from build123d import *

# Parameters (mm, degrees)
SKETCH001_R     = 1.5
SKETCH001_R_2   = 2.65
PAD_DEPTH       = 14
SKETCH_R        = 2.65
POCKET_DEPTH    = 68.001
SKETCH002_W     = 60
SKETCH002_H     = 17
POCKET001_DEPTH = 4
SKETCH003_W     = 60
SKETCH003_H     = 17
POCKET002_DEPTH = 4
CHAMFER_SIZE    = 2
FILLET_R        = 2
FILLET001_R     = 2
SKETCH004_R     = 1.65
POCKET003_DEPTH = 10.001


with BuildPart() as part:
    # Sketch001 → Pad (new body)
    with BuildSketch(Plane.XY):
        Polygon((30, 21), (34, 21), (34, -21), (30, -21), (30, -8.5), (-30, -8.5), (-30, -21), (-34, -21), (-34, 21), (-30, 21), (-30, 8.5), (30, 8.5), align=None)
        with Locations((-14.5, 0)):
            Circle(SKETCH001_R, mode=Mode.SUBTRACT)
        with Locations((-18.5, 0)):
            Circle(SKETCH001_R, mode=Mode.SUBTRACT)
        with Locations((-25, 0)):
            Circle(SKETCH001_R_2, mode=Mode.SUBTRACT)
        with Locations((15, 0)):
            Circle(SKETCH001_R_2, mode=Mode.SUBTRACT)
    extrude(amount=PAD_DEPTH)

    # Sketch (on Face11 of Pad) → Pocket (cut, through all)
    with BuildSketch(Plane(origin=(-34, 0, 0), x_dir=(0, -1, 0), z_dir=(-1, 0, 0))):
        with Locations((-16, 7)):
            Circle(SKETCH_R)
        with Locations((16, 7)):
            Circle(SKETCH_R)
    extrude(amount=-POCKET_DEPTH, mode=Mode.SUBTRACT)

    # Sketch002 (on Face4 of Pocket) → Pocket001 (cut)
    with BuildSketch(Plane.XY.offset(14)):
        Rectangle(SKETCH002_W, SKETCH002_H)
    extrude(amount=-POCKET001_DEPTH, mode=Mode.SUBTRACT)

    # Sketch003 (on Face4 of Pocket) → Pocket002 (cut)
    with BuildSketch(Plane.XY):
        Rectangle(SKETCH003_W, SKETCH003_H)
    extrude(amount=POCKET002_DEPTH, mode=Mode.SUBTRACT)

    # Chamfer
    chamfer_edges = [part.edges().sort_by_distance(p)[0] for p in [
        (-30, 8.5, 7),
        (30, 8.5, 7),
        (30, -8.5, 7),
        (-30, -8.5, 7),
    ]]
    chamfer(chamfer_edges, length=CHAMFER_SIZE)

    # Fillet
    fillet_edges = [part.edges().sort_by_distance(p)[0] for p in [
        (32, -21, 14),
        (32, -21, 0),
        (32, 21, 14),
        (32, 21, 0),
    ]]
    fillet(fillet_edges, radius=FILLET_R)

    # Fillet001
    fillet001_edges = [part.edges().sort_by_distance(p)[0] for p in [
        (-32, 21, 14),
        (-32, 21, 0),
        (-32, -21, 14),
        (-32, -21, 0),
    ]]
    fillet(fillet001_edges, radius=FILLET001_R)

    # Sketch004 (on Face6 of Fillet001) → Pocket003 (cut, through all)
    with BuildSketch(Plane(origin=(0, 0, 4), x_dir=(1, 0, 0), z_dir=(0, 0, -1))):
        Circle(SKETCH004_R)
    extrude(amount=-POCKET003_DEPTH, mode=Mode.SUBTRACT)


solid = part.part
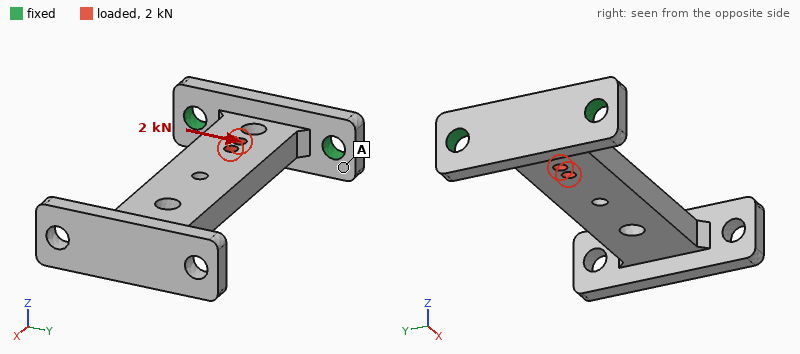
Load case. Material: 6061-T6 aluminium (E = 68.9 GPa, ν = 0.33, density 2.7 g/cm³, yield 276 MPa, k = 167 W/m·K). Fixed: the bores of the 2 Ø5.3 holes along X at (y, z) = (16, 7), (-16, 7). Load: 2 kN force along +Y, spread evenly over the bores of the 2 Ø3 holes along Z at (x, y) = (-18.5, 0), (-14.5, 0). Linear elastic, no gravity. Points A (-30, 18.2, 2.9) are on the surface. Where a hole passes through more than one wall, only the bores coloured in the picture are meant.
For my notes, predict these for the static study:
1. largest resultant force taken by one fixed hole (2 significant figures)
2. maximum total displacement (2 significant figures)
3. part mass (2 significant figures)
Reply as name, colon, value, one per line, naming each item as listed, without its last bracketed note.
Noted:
largest resultant force taken by one fixed hole: 1.6 kN
maximum total displacement: 0.17 mm
part mass: 27 g
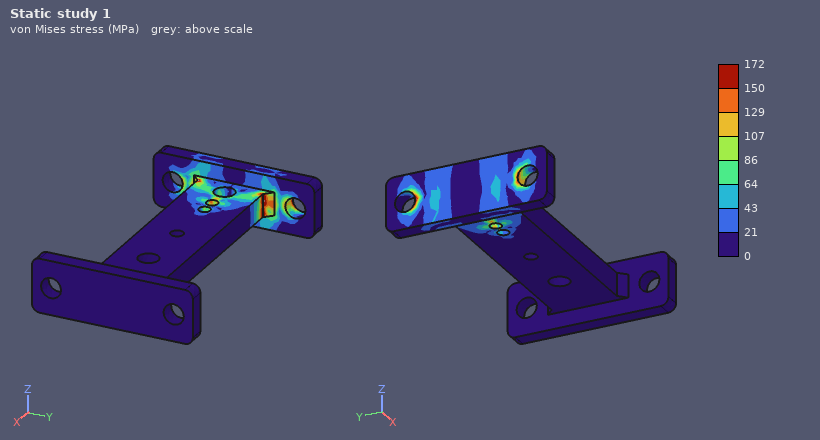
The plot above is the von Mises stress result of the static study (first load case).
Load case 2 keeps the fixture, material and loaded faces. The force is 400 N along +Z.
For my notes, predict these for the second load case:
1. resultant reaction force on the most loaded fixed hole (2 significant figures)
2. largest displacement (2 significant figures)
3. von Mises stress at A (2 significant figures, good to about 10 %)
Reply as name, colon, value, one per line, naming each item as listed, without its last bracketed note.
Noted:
resultant reaction force on the most loaded fixed hole: 200 N
largest displacement: 0.33 mm
von Mises stress at A: 13 MPa
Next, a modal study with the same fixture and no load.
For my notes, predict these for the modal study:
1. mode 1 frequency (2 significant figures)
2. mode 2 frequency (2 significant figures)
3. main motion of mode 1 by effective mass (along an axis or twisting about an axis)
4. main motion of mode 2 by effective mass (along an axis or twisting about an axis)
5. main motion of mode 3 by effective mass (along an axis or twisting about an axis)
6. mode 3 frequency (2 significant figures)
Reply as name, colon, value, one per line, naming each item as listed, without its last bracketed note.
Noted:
mode 1 frequency: 630 Hz
mode 2 frequency: 1900 Hz
main motion of mode 1 by effective mass: along Z
main motion of mode 2 by effective mass: along Y
main motion of mode 3 by effective mass: twisting about X
mode 3 frequency: 2900 Hz
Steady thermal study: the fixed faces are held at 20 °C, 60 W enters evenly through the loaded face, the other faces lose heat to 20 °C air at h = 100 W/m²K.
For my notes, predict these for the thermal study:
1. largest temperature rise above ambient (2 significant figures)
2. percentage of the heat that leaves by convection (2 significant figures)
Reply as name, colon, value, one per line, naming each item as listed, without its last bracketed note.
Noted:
largest temperature rise above ambient: 70 K
percentage of the heat that leaves by convection: 32 %
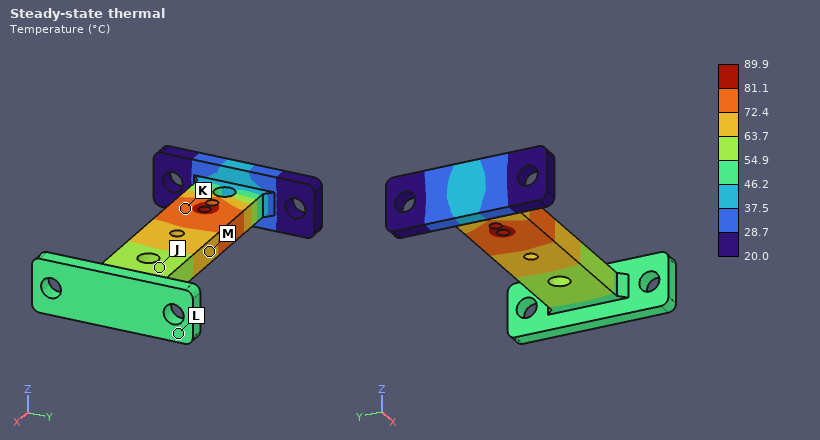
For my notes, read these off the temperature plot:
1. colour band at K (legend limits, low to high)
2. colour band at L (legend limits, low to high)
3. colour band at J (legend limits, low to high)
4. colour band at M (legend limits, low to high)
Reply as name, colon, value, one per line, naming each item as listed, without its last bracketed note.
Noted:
colour band at K: 72.4 to 81.1 °C
colour band at L: 46.2 to 54.9 °C
colour band at J: 54.9 to 63.7 °C
colour band at M: 63.7 to 72.4 °C
